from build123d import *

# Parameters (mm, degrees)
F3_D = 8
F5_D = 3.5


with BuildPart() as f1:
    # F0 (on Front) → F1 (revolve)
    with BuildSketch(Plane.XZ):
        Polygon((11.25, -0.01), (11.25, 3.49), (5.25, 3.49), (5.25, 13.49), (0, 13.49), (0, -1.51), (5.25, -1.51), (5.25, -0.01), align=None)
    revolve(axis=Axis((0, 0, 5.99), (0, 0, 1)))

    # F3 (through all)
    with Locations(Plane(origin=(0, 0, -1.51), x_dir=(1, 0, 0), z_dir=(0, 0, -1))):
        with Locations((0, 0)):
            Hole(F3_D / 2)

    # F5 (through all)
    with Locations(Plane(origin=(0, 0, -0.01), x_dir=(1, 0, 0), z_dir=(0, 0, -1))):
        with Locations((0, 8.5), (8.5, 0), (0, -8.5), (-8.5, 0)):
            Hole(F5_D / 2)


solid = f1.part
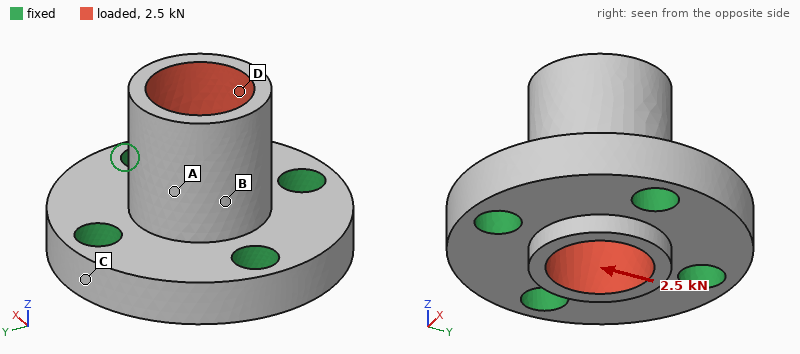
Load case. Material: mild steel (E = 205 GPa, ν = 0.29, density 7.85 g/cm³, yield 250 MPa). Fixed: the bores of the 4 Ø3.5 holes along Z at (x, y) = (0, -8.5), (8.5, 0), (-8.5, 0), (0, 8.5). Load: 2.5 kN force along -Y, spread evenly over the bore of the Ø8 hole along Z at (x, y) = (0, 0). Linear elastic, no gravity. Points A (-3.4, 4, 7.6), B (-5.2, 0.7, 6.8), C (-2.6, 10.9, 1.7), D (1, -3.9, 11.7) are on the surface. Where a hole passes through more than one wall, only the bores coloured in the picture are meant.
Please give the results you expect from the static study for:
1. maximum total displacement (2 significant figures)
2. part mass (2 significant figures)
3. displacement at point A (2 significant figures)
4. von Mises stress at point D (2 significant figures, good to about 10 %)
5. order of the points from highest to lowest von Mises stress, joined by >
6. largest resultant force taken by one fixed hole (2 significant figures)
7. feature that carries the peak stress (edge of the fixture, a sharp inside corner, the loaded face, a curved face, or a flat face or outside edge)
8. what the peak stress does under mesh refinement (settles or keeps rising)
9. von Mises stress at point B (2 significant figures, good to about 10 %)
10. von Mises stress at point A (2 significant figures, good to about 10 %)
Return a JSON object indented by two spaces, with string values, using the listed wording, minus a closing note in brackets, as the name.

{
  "maximum total displacement": "13 µm",
  "part mass": "12 g",
  "displacement at point A": "7.1 µm",
  "von Mises stress at point D": "31 MPa",
  "order of the points from highest to lowest von Mises stress, joined by >": "B > A > D > C",
  "largest resultant force taken by one fixed hole": "1.0 kN",
  "feature that carries the peak stress": "a sharp inside corner",
  "what the peak stress does under mesh refinement": "keeps rising",
  "von Mises stress at point B": "84 MPa",
  "von Mises stress at point A": "57 MPa"
}
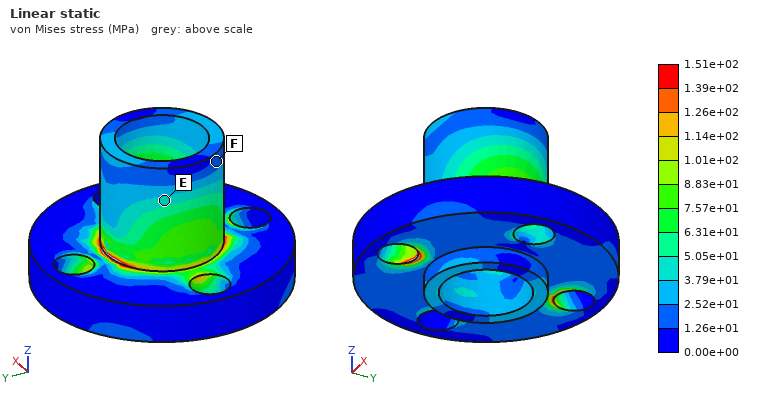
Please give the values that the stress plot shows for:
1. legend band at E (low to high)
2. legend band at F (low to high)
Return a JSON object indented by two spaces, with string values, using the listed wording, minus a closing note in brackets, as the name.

{
  "legend band at E": "3.79e+01 to 5.05e+01 MPa",
  "legend band at F": "1.26e+01 to 2.52e+01 MPa"
}
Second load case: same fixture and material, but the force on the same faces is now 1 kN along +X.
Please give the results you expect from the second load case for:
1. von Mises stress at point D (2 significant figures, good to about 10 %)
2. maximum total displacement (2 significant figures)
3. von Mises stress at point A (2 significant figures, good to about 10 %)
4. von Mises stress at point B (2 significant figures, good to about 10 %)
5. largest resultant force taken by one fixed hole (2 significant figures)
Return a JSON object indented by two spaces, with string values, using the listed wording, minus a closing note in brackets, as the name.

{
  "von Mises stress at point D": "14 MPa",
  "maximum total displacement": "5.3 µm",
  "von Mises stress at point A": "26 MPa",
  "von Mises stress at point B": "14 MPa",
  "largest resultant force taken by one fixed hole": "410 N"
}
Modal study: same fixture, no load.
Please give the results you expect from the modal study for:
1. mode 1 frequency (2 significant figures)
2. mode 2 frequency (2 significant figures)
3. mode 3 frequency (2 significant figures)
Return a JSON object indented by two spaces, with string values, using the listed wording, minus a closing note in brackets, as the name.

{
  "mode 1 frequency": "39 kHz",
  "mode 2 frequency": "39 kHz",
  "mode 3 frequency": "45 kHz"
}
